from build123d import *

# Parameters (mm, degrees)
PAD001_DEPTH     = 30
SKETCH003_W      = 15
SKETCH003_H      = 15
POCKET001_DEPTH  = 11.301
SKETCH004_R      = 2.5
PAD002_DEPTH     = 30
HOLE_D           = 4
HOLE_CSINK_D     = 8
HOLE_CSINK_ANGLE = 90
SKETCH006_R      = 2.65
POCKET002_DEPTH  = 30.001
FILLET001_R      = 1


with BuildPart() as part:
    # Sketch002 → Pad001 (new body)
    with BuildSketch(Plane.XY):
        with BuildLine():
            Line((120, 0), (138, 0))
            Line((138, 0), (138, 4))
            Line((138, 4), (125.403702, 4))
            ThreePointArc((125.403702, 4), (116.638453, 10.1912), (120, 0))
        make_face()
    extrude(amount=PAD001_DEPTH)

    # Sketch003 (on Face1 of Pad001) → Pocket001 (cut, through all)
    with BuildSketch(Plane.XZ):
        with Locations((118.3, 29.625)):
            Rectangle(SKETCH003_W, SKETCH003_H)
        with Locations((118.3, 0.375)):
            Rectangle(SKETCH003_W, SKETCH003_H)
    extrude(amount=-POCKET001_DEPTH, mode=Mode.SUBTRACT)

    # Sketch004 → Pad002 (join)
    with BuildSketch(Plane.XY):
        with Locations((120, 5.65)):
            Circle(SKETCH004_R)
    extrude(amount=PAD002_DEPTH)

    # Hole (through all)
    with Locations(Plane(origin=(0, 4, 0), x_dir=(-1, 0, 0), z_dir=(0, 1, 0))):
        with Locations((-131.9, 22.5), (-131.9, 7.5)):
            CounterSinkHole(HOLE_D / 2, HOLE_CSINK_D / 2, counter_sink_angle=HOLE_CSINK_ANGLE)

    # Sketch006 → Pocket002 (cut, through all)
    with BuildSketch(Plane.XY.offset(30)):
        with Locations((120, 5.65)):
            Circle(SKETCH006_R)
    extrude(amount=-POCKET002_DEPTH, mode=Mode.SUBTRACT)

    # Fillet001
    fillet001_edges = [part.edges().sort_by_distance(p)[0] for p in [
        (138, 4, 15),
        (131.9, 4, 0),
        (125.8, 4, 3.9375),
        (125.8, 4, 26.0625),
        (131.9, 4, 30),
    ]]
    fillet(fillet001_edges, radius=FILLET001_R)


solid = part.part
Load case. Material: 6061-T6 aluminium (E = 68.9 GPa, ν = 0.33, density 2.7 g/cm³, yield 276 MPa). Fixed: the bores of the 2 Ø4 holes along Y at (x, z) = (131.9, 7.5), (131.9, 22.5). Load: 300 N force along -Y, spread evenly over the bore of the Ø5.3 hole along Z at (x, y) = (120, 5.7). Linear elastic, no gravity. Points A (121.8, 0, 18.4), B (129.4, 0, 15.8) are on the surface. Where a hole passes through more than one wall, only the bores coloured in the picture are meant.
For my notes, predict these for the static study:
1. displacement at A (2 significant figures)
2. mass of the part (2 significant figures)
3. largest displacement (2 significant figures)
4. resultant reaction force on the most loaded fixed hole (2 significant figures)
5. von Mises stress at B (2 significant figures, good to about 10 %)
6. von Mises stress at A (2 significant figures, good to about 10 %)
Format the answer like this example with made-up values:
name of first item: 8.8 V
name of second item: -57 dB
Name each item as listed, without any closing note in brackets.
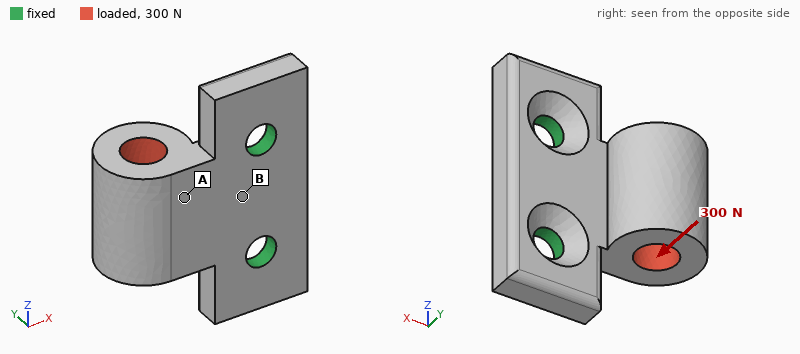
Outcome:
displacement at A: 32 µm
mass of the part: 6.8 g
largest displacement: 68 µm
resultant reaction force on the most loaded fixed hole: 170 N
von Mises stress at B: 41 MPa
von Mises stress at A: 16 MPa
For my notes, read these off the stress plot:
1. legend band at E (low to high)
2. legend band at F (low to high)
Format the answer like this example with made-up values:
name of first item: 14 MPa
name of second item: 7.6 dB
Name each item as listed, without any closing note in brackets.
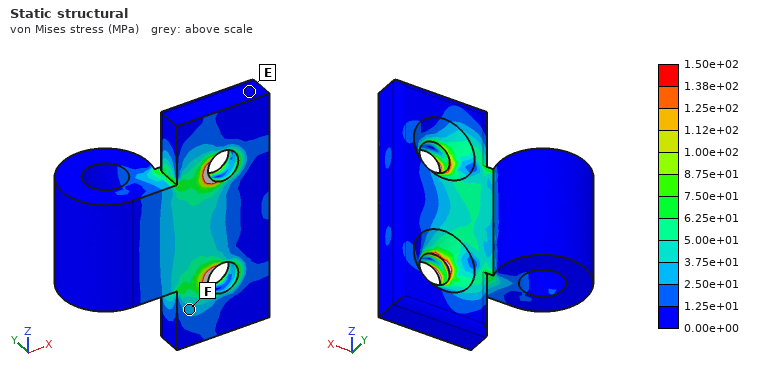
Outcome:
legend band at E: 0.00e+00 to 1.25e+01 MPa
legend band at F: 2.50e+01 to 3.75e+01 MPa
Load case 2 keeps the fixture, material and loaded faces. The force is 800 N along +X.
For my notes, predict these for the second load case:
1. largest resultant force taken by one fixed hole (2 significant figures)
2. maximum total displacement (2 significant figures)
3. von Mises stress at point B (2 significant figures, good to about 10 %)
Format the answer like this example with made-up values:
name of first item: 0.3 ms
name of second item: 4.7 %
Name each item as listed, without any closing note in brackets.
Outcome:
largest resultant force taken by one fixed hole: 410 N
maximum total displacement: 85 µm
von Mises stress at point B: 44 MPa
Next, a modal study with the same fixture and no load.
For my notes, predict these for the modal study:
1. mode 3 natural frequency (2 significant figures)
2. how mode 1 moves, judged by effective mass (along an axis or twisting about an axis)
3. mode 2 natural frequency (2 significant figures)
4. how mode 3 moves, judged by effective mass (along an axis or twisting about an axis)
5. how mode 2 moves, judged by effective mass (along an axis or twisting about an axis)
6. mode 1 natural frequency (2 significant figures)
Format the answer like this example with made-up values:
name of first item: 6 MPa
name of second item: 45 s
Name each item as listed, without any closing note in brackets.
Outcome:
mode 3 natural frequency: 29 kHz
how mode 1 moves, judged by effective mass: along Y
mode 2 natural frequency: 20 kHz
how mode 3 moves, judged by effective mass: along Z
how mode 2 moves, judged by effective mass: along Z
mode 1 natural frequency: 6500 Hz
